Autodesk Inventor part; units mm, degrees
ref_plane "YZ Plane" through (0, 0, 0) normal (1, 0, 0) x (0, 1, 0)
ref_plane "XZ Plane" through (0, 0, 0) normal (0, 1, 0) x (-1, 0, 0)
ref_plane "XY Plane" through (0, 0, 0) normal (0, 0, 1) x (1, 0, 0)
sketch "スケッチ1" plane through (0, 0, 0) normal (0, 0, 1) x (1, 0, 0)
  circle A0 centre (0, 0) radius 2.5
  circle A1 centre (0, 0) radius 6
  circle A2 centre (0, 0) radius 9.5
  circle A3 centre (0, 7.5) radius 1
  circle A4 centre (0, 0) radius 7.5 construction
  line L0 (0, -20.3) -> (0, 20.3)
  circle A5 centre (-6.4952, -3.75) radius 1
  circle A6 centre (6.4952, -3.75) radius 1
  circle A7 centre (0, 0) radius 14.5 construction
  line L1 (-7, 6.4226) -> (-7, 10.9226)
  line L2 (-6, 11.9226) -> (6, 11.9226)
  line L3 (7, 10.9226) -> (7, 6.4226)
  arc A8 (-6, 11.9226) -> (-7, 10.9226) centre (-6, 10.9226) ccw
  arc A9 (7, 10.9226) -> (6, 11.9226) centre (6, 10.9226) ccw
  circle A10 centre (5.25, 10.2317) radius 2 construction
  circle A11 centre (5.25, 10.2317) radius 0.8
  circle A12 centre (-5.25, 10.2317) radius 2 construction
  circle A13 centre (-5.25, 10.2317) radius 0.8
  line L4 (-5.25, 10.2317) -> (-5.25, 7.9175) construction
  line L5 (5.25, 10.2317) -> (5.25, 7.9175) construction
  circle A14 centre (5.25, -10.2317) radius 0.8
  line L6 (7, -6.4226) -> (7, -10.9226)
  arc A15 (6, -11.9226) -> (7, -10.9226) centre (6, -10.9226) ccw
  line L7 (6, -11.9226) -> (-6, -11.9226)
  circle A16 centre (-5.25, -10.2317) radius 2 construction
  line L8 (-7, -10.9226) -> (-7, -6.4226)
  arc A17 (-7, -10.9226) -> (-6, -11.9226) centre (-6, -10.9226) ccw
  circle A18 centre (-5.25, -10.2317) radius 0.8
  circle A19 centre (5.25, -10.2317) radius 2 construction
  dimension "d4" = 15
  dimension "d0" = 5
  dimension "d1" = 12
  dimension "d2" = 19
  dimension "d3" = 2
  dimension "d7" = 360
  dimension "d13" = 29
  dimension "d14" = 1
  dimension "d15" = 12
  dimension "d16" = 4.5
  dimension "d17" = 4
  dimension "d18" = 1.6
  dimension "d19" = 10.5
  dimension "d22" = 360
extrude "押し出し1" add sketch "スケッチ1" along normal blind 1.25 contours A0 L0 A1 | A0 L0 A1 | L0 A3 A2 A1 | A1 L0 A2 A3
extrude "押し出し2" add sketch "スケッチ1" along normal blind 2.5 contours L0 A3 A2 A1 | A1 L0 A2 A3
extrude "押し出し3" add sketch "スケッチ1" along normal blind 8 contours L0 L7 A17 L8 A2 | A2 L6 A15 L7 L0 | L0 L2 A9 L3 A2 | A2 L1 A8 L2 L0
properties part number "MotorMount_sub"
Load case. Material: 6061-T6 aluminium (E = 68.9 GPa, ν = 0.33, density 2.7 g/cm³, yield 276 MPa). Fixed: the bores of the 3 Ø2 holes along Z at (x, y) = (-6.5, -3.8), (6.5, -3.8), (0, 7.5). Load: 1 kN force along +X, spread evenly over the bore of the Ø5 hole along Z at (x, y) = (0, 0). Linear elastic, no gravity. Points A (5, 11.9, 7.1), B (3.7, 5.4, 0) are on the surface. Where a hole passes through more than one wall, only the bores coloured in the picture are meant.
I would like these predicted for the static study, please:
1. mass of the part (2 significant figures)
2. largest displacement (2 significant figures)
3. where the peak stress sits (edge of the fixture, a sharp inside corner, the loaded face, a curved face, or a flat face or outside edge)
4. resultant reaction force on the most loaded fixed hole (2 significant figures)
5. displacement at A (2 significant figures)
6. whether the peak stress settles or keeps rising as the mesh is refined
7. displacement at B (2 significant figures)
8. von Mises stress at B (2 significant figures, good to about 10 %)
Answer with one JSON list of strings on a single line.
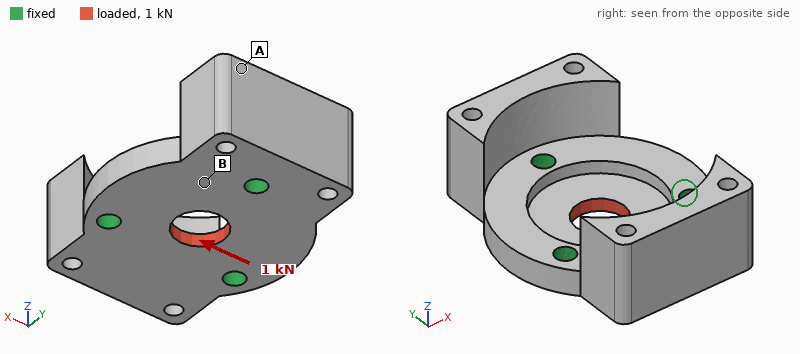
["3.2 g", "5.7 µm", "edge of the fixture", "350 N", "2.4 µm", "keeps rising", "2.5 µm", "29 MPa"]
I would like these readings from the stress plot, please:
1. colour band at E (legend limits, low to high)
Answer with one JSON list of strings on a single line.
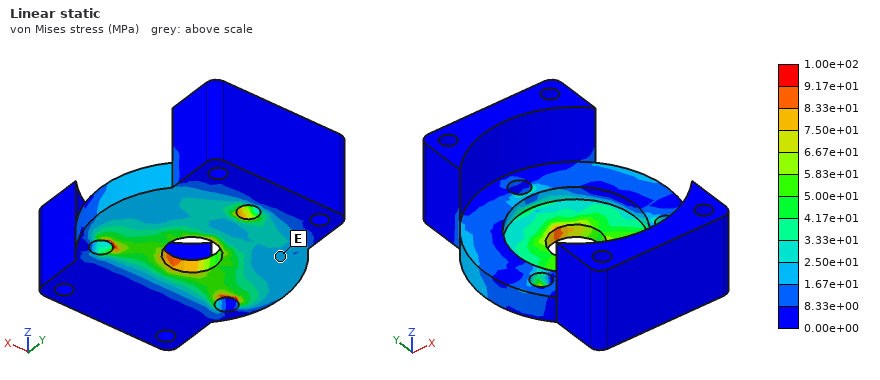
["1.67e+01 to 2.50e+01 MPa"]
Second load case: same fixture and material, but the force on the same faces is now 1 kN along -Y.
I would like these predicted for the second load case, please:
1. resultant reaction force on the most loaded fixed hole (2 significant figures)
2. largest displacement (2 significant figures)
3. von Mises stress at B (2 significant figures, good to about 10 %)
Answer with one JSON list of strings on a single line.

["340 N", "5.7 µm", "21 MPa"]
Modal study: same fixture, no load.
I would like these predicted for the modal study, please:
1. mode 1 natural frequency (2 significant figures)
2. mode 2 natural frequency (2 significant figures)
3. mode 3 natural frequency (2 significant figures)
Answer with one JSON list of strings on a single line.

["12 kHz", "22 kHz", "25 kHz"]
